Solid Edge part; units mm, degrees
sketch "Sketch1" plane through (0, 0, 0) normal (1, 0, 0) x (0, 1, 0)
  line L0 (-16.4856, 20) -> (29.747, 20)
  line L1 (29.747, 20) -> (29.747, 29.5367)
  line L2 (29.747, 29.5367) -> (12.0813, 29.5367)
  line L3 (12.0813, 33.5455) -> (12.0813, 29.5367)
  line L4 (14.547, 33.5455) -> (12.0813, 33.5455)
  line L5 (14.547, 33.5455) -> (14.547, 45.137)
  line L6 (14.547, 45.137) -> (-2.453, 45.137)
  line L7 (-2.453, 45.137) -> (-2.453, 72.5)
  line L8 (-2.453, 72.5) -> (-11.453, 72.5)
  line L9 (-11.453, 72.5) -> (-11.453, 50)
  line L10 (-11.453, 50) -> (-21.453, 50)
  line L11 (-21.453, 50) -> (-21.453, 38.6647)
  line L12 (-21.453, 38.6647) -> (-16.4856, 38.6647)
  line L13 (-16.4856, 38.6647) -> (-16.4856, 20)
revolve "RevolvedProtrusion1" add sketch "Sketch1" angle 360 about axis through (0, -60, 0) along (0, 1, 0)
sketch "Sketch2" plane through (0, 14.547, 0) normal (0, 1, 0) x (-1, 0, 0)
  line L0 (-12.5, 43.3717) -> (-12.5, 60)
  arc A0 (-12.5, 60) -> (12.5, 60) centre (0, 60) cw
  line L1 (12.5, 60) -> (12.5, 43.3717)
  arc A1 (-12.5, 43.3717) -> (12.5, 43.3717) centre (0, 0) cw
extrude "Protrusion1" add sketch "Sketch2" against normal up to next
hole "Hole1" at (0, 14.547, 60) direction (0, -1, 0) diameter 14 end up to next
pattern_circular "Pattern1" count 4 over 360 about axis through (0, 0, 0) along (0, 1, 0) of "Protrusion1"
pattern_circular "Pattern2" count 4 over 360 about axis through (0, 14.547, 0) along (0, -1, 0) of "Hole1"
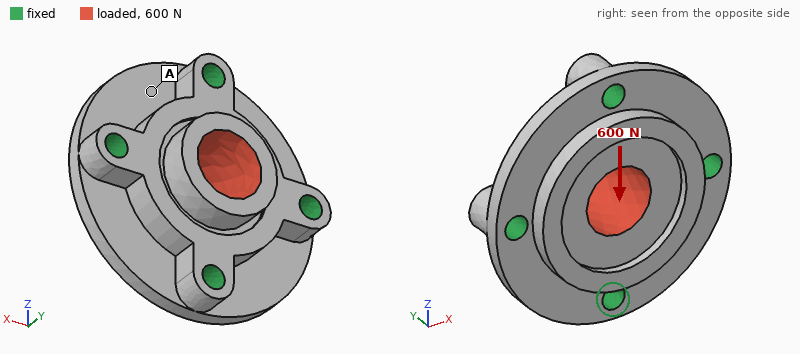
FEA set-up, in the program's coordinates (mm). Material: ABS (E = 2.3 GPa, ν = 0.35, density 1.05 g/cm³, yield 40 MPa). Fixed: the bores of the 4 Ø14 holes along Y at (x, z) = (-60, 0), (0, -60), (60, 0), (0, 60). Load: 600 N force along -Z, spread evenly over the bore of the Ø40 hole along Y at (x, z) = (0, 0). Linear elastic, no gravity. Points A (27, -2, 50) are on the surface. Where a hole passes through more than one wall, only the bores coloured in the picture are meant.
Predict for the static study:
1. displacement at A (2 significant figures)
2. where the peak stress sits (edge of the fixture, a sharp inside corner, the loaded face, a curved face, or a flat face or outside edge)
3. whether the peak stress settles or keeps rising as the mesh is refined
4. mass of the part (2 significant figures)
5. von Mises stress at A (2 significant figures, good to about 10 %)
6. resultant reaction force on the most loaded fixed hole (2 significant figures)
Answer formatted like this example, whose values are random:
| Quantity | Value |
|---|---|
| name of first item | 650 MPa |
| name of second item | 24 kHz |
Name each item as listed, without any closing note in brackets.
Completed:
| Quantity | Value |
|---|---|
| displacement at A | 2.8 µm |
| where the peak stress sits | edge of the fixture |
| whether the peak stress settles or keeps rising as the mesh is refined | keeps rising |
| mass of the part | 340 g |
| von Mises stress at A | 0.079 MPa |
| resultant reaction force on the most loaded fixed hole | 210 N |
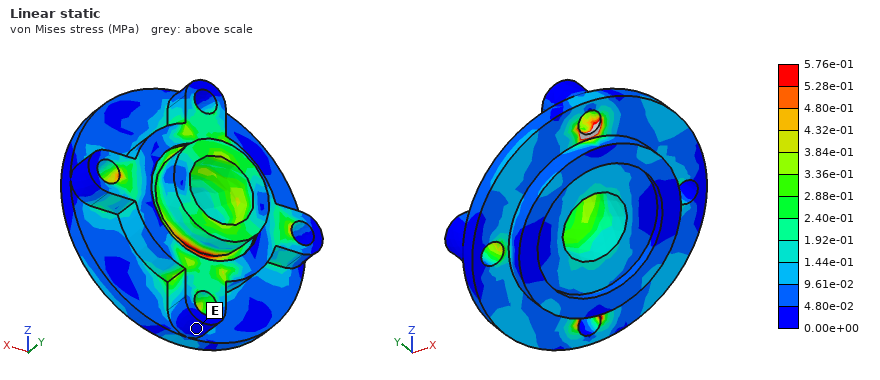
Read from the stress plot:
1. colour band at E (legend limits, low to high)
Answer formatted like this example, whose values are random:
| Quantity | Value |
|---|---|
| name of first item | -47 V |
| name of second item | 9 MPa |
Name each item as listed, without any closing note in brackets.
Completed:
| Quantity | Value |
|---|---|
| colour band at E | 0.00e+00 to 4.80e-02 MPa |
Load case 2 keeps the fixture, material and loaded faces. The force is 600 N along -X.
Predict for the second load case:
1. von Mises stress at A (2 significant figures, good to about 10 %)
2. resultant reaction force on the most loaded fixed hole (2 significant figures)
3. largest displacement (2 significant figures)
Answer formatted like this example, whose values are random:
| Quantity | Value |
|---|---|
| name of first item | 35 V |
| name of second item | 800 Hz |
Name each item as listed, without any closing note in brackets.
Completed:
| Quantity | Value |
|---|---|
| von Mises stress at A | 0.081 MPa |
| resultant reaction force on the most loaded fixed hole | 210 N |
| largest displacement | 11 µm |
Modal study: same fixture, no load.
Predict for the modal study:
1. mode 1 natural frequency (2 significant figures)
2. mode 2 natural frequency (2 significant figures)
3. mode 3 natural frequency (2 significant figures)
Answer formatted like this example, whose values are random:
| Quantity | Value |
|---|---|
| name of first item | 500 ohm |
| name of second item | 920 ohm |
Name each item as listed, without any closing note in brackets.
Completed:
| Quantity | Value |
|---|---|
| mode 1 natural frequency | 2600 Hz |
| mode 2 natural frequency | 2700 Hz |
| mode 3 natural frequency | 2700 Hz |
